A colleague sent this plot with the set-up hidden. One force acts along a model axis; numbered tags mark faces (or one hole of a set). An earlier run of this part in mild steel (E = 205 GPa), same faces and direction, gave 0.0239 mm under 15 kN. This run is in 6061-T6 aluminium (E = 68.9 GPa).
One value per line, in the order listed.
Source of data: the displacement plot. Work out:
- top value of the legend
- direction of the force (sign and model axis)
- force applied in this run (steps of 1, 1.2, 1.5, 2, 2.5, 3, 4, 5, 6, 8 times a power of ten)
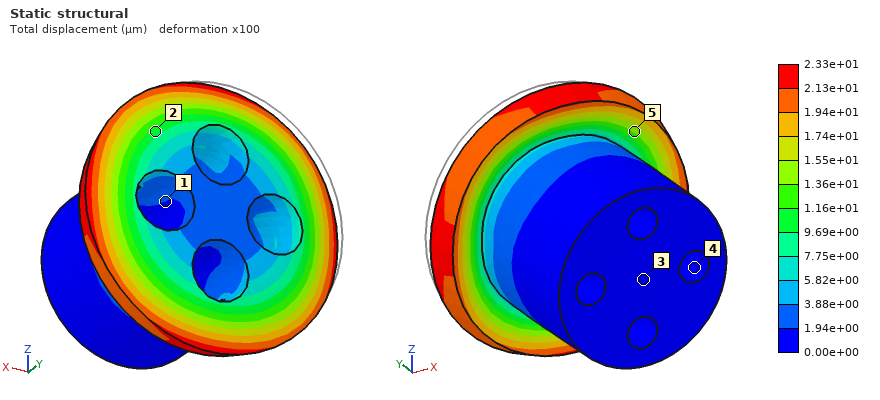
2.33e+01 µm
-Y
5 kN
